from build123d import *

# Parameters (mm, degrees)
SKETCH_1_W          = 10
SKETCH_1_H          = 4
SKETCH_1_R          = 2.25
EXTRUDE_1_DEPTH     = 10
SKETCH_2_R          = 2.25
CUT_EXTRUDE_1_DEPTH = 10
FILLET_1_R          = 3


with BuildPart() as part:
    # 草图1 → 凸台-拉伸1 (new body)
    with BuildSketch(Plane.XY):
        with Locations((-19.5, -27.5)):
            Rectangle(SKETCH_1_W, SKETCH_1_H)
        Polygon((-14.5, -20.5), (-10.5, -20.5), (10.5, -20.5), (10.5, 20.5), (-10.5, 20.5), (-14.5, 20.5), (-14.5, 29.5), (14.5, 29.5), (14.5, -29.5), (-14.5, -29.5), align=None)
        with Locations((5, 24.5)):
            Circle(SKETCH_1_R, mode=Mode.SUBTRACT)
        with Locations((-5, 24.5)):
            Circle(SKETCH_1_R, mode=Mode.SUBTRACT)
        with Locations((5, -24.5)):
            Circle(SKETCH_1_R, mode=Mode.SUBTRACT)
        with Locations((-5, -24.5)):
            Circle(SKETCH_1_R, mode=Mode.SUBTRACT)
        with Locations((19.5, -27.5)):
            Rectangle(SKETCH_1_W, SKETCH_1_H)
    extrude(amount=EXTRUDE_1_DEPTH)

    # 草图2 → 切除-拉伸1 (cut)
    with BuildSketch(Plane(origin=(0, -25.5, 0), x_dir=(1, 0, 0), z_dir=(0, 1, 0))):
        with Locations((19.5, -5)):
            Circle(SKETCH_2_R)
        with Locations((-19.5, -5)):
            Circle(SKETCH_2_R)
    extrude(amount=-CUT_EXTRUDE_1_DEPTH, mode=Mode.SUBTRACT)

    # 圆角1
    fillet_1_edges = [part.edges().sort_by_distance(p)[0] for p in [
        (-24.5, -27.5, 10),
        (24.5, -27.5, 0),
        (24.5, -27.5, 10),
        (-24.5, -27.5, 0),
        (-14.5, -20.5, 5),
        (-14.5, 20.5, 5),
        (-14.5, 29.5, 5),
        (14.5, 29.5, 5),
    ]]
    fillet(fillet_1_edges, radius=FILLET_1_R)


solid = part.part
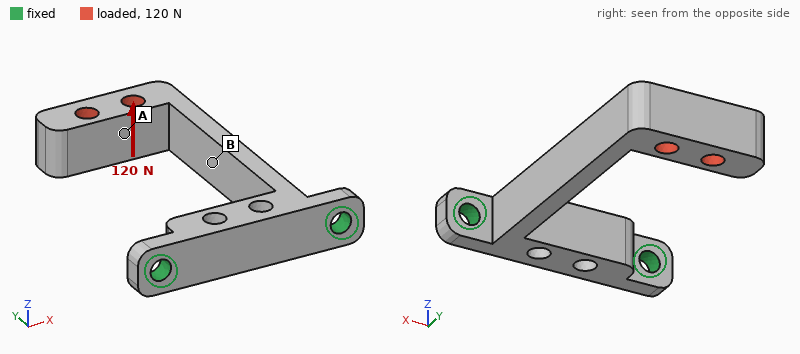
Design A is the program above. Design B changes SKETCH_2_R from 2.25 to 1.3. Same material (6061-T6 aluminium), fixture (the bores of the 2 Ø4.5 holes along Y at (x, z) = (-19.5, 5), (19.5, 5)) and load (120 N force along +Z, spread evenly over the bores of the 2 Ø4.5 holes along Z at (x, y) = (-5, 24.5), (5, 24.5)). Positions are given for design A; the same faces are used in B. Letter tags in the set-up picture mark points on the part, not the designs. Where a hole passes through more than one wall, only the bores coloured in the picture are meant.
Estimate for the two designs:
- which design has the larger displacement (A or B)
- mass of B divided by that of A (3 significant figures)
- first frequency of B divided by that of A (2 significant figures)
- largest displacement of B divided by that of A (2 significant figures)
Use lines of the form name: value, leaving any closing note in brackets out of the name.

which design has the larger displacement: B
mass of B divided by that of A: 1.01
first frequency of B divided by that of A: 1.00
largest displacement of B divided by that of A: 1.1
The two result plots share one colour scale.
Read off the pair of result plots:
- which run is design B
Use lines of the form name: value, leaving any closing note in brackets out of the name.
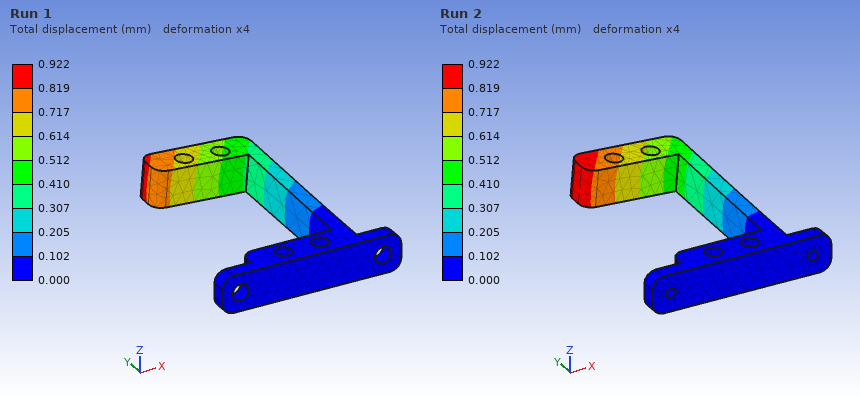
which run is design B: Run 2
